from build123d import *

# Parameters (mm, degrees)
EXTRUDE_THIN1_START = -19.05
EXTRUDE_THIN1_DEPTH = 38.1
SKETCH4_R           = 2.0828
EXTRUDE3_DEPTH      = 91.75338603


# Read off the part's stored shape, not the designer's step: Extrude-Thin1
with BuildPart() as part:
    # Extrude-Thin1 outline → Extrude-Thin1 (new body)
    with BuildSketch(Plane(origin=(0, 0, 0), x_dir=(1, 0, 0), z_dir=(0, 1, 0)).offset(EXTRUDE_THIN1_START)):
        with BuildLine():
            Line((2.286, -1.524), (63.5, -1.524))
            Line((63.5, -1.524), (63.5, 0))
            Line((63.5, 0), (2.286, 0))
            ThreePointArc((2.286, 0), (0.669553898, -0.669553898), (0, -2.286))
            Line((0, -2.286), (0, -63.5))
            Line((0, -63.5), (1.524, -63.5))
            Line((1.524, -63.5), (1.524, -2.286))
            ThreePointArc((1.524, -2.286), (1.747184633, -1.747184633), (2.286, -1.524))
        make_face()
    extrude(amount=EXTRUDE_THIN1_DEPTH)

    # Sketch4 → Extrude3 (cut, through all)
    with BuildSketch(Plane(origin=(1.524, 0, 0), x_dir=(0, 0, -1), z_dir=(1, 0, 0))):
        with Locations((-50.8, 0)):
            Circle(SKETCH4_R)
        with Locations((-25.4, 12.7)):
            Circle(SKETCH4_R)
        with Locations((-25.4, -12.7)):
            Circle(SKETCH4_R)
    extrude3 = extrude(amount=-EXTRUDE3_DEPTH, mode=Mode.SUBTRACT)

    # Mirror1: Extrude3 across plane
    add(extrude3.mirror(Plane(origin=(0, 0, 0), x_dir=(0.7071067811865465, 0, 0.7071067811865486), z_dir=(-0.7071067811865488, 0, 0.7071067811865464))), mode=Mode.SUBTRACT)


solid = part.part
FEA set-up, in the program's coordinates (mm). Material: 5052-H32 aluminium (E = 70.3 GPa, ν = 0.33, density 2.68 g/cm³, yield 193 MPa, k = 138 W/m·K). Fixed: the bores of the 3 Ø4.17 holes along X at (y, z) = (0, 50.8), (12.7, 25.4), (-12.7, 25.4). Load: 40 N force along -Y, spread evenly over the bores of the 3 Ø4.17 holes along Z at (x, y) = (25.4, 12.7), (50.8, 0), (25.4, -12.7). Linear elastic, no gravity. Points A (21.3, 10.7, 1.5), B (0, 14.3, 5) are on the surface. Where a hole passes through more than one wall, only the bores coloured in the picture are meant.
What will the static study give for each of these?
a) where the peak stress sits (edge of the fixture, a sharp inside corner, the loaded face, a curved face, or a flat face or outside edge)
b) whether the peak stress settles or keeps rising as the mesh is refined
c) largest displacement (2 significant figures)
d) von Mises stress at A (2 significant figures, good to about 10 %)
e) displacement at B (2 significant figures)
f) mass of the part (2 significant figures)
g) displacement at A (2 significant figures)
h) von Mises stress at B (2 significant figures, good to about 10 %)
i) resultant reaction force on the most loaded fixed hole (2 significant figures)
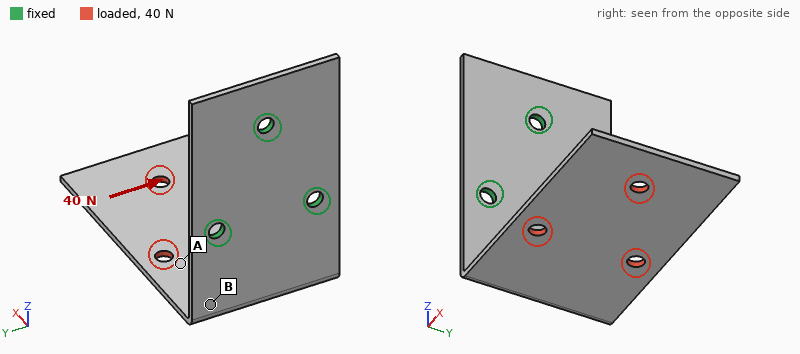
edge of the fixture
keeps rising
0.84 mm
8.1 MPa
0.15 mm
19 g
0.30 mm
45 MPa
62 N
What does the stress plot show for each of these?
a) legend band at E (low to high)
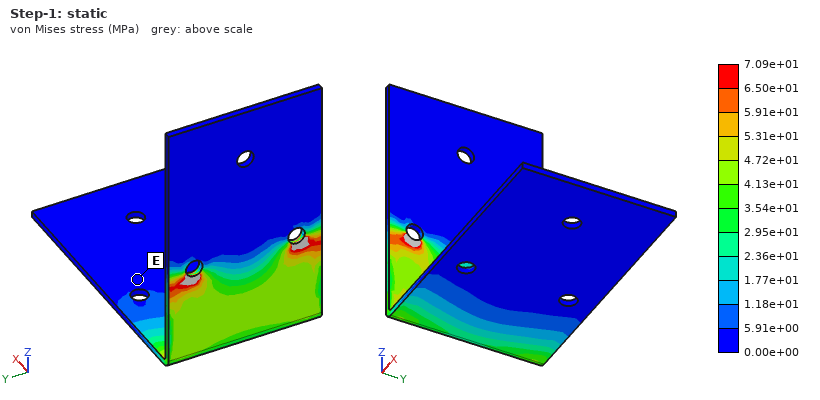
0.00e+00 to 5.91e+00 MPa
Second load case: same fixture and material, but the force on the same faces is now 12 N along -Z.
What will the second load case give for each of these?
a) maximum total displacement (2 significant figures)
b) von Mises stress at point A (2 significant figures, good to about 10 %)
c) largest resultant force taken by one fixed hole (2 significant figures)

1.1 mm
9.0 MPa
5.8 N
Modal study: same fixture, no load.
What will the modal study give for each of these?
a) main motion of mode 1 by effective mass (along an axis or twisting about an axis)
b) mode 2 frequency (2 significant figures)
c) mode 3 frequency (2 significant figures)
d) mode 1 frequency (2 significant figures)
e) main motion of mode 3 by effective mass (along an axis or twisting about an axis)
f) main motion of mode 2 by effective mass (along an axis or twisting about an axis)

along Z
430 Hz
870 Hz
210 Hz
along X
along Y
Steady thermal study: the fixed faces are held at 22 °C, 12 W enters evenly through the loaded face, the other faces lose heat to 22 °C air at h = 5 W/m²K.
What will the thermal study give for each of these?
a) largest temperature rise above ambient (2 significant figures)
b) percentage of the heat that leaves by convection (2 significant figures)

81 K
14 %
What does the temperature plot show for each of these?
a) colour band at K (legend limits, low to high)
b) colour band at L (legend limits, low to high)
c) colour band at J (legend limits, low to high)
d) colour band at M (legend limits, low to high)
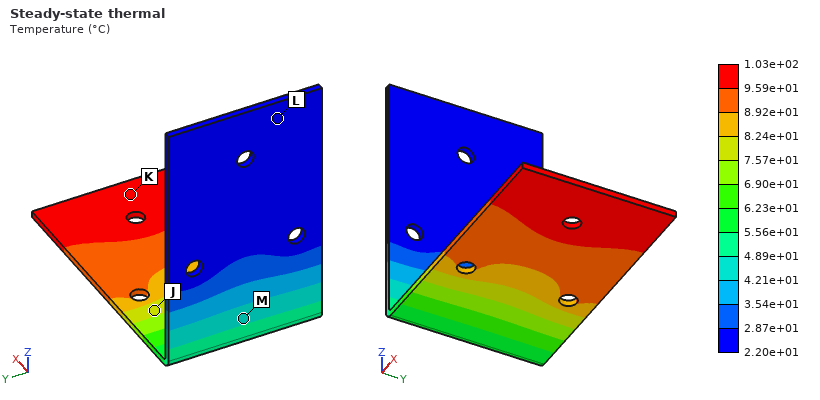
9.59e+01 to 1.03e+02 °C
2.20e+01 to 2.87e+01 °C
7.57e+01 to 8.24e+01 °C
4.21e+01 to 4.89e+01 °C
